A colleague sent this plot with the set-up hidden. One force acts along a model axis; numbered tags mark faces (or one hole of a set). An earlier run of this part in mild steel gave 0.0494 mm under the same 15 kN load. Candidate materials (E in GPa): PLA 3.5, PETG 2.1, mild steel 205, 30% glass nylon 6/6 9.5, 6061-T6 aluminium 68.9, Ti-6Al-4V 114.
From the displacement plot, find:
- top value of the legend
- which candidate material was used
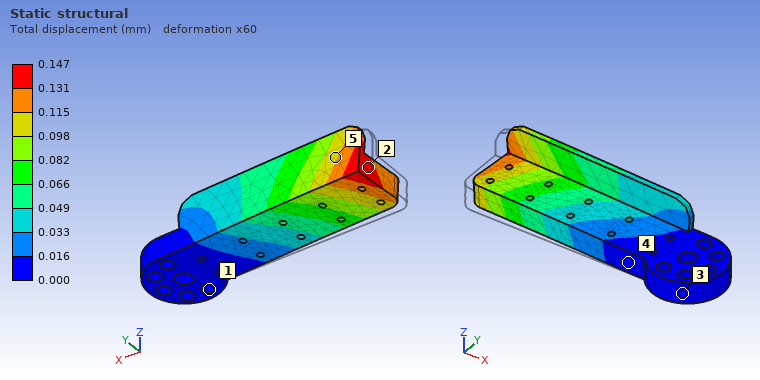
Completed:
0.147 mm
6061-T6 aluminium
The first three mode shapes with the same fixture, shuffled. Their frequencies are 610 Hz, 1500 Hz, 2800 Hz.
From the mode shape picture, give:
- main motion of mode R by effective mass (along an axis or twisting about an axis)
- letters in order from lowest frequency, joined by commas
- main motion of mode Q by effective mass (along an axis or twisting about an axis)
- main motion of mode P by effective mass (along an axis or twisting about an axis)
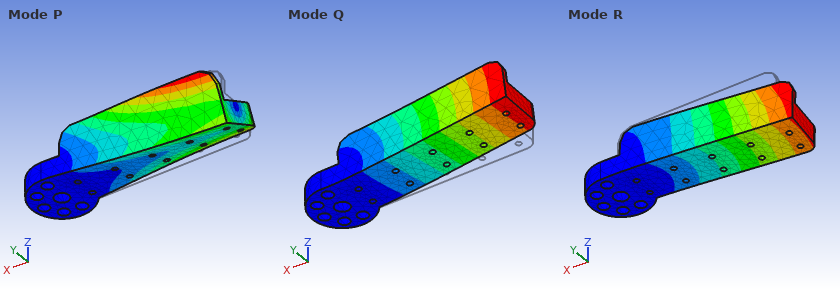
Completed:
along Y
Q, R, P
along Z
twisting about X
